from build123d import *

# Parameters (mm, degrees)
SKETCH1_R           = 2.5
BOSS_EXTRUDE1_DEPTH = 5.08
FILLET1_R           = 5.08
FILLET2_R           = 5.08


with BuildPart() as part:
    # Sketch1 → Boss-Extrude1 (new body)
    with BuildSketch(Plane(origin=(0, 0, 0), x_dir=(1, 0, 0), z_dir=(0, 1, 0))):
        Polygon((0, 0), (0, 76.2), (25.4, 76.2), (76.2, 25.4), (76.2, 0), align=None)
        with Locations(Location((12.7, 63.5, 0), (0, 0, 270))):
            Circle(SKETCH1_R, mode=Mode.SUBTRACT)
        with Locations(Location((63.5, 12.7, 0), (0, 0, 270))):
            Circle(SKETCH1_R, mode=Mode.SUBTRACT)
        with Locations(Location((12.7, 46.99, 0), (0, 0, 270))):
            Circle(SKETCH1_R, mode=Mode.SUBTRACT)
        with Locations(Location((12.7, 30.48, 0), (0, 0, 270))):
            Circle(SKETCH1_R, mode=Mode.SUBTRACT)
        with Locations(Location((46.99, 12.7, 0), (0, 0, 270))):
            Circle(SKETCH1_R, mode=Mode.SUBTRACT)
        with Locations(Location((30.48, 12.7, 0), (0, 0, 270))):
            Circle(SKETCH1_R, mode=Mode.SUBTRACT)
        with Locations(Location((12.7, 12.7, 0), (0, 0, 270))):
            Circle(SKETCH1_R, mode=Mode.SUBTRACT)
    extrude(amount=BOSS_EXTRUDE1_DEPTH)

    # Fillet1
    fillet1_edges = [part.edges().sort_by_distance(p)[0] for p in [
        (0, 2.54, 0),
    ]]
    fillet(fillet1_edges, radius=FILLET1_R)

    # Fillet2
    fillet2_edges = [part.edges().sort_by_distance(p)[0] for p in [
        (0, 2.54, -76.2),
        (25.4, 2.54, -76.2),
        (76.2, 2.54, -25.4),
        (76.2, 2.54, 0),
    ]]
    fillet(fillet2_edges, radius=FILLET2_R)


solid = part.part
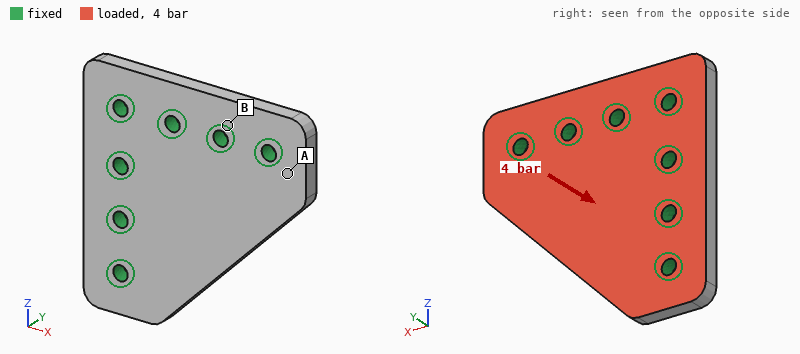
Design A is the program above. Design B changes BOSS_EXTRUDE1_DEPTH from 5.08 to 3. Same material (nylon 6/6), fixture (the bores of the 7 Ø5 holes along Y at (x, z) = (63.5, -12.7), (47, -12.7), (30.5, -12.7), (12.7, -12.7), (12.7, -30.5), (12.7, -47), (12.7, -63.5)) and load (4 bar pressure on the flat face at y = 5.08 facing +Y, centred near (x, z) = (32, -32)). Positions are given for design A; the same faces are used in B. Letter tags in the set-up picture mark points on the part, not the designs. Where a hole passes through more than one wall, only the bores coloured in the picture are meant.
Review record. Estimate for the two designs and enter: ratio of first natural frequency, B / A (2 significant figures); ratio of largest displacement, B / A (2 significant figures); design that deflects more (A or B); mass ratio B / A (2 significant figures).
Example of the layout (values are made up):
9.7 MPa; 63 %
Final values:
0.62; 4.5; B; 0.59
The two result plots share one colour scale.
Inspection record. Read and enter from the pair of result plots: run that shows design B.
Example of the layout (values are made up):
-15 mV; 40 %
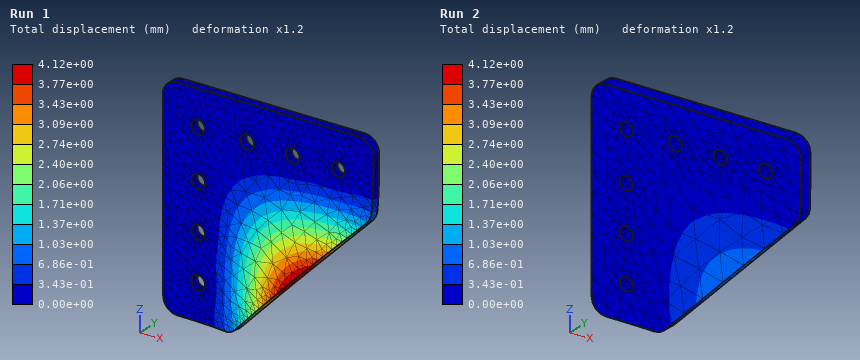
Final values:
Run 1
